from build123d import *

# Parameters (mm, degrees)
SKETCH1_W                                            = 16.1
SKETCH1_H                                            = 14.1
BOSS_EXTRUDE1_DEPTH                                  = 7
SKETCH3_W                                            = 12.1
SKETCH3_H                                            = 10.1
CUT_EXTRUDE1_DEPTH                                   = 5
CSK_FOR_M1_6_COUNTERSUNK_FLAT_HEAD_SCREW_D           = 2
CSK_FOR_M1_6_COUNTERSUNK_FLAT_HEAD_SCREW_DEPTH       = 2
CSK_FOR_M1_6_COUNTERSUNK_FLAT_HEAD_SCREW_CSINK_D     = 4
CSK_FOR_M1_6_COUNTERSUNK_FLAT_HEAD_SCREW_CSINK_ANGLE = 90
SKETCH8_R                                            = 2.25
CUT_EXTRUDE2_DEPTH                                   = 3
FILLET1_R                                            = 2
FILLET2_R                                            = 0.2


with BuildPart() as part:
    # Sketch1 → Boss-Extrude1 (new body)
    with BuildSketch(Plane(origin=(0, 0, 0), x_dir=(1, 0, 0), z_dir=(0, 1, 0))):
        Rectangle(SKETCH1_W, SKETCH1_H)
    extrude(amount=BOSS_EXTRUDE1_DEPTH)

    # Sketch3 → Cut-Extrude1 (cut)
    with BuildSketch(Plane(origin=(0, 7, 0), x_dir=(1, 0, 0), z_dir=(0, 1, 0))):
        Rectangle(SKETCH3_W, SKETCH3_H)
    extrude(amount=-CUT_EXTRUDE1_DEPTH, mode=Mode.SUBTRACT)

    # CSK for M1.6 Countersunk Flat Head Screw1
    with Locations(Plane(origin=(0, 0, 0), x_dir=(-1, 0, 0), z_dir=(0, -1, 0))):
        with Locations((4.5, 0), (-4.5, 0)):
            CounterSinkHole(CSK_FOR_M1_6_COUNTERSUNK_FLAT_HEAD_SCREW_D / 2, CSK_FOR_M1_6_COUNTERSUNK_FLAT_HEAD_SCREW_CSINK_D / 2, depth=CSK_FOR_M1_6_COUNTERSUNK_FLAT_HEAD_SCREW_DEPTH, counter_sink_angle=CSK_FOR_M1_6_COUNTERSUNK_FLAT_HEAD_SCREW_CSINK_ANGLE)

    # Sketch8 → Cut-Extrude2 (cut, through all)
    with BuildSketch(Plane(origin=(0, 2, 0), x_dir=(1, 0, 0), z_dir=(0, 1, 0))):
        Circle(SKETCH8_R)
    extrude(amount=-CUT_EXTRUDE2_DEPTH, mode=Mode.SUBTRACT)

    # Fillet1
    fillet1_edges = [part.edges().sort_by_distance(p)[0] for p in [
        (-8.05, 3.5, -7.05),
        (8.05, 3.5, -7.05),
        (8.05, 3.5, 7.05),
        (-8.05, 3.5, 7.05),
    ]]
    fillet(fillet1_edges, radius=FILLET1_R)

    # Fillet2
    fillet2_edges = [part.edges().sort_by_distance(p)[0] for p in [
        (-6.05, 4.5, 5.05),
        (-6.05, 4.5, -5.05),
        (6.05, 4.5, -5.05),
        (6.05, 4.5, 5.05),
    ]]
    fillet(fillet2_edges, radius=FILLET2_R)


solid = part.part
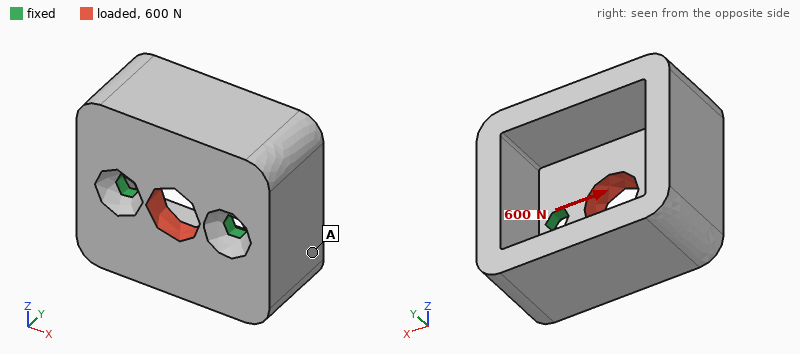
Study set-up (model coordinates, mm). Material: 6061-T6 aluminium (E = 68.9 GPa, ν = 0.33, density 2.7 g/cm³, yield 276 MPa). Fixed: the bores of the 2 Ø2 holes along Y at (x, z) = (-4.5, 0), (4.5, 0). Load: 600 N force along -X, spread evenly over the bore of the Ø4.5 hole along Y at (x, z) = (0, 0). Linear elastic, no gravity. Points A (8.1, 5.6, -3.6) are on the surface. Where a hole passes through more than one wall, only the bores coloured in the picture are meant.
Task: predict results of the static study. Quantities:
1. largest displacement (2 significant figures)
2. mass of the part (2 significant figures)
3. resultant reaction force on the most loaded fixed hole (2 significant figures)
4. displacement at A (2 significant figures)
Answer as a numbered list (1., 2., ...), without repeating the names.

1. 2.2 µm
2. 2.4 g
3. 300 N
4. 0.74 µm
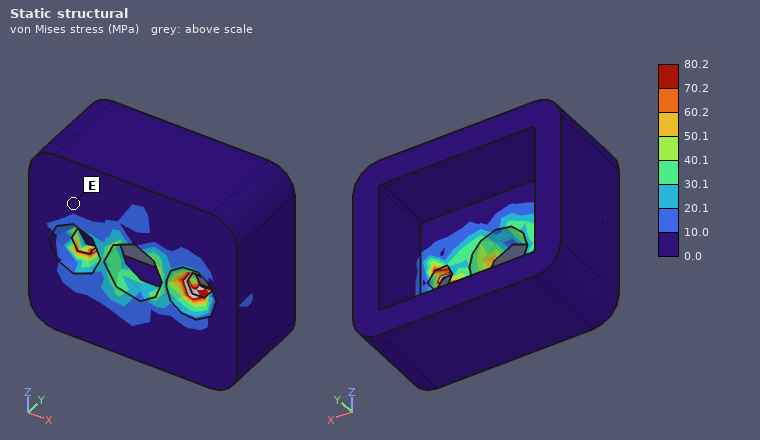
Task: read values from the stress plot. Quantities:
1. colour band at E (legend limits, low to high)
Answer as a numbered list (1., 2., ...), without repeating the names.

1. 0.0 to 10.0 MPa
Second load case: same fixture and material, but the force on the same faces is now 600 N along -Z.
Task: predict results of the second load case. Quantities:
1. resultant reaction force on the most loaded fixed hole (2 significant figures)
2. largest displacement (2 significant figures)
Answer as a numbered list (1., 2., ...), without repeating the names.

1. 300 N
2. 5.9 µm
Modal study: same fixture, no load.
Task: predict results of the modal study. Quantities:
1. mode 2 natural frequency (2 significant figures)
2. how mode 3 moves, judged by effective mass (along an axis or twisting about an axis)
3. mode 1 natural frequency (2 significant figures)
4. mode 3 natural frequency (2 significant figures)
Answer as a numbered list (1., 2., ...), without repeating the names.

1. 24 kHz
2. along X
3. 11 kHz
4. 28 kHz
